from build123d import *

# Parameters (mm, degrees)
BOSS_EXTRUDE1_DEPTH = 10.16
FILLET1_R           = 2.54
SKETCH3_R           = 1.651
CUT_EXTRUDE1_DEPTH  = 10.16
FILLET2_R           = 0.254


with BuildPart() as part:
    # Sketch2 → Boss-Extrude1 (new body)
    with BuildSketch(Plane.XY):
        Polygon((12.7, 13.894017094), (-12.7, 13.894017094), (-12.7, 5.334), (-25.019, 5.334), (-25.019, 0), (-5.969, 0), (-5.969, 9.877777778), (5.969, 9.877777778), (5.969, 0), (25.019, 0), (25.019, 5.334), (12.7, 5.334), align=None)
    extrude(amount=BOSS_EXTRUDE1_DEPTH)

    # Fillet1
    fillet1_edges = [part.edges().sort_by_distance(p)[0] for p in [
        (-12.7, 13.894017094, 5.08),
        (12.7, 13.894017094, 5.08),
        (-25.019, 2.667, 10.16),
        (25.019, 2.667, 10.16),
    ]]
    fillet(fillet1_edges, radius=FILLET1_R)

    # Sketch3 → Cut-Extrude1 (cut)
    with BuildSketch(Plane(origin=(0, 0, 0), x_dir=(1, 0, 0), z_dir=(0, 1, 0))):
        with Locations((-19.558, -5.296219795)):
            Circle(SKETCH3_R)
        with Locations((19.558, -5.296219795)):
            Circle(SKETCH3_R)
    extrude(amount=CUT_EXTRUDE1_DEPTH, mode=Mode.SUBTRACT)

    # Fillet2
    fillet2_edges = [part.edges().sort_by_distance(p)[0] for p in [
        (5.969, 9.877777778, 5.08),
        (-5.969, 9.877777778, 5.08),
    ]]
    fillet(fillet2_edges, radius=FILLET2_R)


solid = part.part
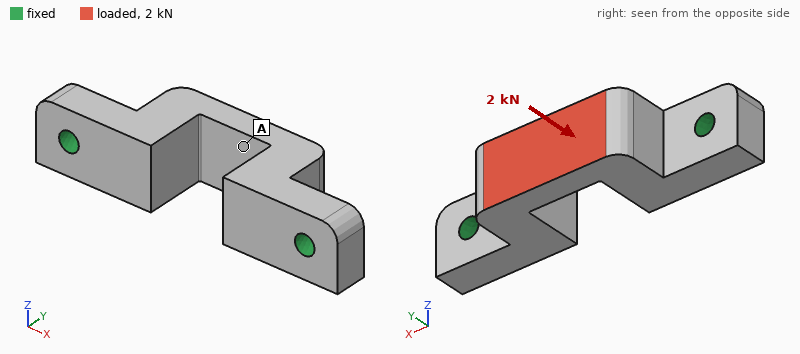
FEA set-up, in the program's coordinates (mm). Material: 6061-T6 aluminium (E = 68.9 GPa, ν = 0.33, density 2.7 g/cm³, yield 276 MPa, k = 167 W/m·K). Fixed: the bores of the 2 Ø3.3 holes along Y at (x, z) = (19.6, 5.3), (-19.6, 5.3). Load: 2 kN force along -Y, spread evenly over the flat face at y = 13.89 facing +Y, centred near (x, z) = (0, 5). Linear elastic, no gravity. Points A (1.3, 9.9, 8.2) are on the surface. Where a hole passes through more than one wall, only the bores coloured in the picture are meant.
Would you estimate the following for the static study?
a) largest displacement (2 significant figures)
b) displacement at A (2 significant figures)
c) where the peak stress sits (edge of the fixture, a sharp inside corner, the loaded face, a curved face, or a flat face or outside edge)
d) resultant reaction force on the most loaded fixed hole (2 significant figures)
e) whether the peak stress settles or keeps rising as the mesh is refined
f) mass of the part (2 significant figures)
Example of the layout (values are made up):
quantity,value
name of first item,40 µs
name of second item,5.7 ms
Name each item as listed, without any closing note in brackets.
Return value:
quantity,value
largest displacement,26 µm
displacement at A,24 µm
where the peak stress sits,edge of the fixture
resultant reaction force on the most loaded fixed hole,1.3 kN
whether the peak stress settles or keeps rising as the mesh is refined,keeps rising
mass of the part,9.7 g
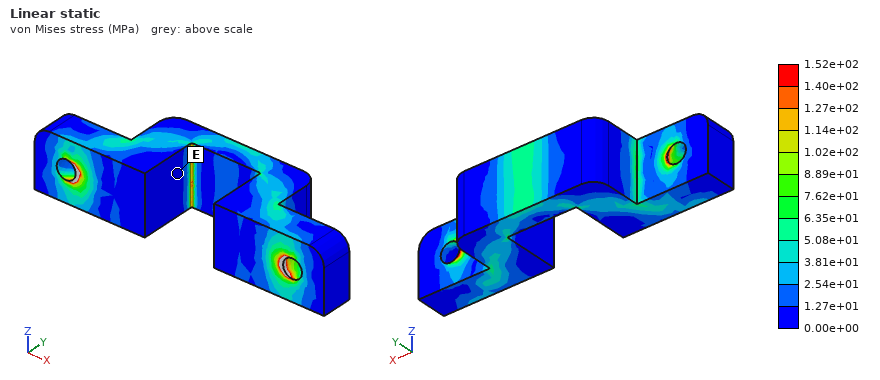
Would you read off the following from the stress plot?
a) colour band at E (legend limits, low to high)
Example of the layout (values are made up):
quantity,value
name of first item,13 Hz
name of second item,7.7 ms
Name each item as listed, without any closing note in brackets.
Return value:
quantity,value
colour band at E,0.00e+00 to 1.27e+01 MPa
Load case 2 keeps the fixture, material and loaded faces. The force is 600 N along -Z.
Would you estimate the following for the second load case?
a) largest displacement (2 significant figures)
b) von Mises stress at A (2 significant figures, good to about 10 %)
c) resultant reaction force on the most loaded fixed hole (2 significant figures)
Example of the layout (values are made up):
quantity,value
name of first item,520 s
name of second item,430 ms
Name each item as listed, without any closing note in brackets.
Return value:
quantity,value
largest displacement,49 µm
von Mises stress at A,17 MPa
resultant reaction force on the most loaded fixed hole,300 N
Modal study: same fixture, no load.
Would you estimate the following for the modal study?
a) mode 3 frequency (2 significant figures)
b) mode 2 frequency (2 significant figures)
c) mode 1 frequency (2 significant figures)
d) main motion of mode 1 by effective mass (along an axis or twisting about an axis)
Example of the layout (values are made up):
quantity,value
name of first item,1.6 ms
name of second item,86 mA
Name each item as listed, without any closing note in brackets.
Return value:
quantity,value
mode 3 frequency,22 kHz
mode 2 frequency,21 kHz
mode 1 frequency,11 kHz
main motion of mode 1 by effective mass,along Z
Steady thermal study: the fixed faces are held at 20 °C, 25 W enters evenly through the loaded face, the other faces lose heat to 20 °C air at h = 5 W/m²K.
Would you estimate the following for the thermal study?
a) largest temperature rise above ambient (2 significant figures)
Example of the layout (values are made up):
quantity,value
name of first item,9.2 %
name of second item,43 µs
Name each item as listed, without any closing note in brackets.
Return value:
quantity,value
largest temperature rise above ambient,26 K
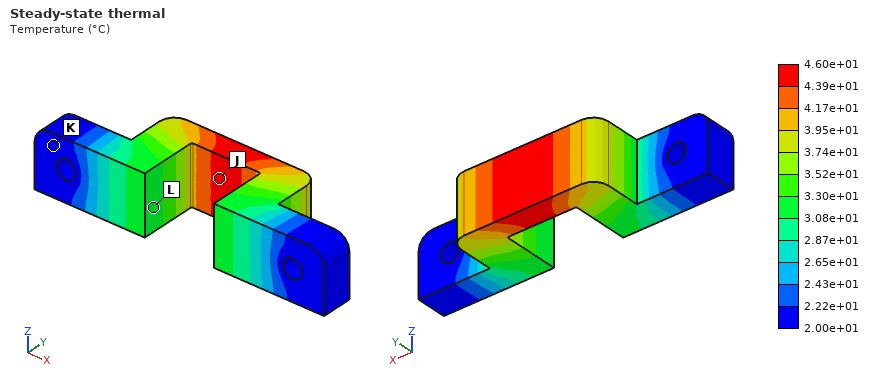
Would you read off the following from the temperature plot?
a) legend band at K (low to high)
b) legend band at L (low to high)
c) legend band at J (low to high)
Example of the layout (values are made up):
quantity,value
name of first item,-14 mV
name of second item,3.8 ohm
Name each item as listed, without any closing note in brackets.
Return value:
quantity,value
legend band at K,2.00e+01 to 2.22e+01 °C
legend band at L,3.08e+01 to 3.30e+01 °C
legend band at J,4.39e+01 to 4.60e+01 °C
